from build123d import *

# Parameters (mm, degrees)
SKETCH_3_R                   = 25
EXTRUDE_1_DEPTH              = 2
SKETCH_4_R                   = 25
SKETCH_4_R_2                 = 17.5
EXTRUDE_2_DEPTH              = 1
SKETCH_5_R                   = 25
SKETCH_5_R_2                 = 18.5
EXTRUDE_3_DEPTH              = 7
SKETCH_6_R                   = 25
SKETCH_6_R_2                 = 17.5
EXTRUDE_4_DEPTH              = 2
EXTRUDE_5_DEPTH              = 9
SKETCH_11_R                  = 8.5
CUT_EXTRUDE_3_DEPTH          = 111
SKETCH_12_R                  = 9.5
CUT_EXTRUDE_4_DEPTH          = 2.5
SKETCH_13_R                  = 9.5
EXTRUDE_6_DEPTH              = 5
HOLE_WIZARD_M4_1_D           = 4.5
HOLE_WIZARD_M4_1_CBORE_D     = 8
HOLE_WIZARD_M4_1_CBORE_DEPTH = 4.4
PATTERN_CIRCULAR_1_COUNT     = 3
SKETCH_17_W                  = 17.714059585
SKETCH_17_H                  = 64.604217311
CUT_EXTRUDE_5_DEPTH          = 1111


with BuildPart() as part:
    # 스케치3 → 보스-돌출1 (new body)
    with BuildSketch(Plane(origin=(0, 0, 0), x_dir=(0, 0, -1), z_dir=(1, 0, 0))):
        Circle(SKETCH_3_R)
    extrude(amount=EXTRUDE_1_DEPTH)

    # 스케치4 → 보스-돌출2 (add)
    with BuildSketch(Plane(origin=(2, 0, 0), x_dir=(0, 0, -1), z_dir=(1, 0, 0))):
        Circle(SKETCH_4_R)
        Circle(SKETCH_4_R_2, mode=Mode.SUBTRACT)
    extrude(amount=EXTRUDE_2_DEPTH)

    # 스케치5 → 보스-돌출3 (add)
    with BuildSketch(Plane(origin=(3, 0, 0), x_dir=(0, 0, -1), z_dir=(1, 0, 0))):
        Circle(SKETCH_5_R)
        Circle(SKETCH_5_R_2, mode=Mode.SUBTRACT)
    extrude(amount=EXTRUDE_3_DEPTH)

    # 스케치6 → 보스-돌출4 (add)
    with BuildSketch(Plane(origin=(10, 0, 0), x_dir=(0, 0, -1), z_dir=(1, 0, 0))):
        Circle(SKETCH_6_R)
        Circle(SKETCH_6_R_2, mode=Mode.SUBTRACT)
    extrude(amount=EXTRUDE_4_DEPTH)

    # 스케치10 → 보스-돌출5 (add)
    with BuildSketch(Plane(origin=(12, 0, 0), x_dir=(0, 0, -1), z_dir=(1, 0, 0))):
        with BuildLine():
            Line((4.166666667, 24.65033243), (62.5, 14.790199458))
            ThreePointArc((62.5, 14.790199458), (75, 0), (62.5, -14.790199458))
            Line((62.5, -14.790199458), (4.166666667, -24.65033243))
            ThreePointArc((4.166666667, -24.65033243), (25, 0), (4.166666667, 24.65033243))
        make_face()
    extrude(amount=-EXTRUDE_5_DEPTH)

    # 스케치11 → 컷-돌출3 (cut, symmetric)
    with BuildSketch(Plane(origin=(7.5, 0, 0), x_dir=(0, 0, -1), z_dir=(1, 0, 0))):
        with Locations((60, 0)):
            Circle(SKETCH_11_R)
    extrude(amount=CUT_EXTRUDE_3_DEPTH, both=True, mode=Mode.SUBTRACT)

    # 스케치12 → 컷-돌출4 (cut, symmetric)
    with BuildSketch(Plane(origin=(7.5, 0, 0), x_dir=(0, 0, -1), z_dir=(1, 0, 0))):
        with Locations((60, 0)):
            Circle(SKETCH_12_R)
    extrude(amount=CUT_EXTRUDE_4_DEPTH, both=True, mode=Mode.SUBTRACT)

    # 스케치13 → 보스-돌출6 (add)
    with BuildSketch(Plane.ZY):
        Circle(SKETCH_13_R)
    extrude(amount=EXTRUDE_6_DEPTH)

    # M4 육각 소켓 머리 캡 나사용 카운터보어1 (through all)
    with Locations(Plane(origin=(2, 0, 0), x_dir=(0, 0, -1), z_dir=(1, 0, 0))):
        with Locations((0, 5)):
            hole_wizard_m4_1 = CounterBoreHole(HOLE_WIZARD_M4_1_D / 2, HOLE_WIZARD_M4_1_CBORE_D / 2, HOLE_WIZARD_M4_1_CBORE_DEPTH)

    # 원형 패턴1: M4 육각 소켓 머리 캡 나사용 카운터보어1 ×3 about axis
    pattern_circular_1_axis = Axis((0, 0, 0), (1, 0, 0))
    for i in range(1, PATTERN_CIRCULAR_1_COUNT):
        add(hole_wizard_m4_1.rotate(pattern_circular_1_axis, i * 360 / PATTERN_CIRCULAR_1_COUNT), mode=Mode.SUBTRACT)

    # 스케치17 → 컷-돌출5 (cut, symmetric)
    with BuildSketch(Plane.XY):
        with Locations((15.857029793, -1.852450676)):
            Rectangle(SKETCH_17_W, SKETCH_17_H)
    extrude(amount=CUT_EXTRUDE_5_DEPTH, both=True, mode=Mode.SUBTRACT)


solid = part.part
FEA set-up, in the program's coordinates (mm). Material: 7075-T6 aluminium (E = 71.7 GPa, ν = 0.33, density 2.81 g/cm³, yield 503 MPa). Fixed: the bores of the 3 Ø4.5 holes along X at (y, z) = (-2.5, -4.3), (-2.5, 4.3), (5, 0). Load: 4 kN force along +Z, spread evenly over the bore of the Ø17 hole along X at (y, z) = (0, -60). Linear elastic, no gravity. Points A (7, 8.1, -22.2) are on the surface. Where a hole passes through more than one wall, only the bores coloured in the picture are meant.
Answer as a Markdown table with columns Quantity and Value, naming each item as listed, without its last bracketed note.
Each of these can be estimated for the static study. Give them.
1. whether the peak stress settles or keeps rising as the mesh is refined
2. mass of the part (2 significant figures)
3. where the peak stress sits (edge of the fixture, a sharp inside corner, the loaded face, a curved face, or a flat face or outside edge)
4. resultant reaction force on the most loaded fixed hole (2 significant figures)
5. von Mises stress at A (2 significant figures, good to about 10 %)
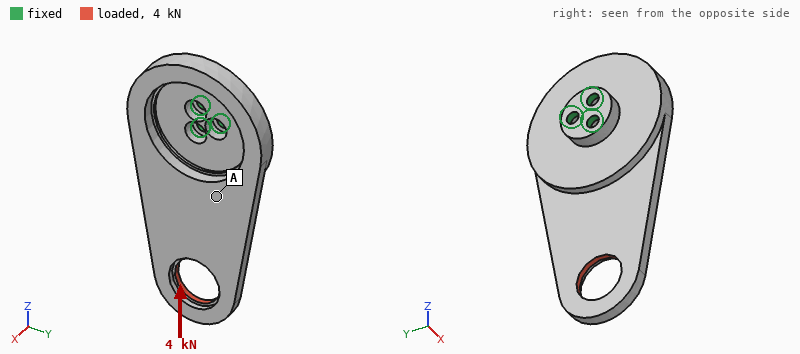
| Quantity | Value |
|---|---|
| whether the peak stress settles or keeps rising as the mesh is refined | keeps rising |
| mass of the part | 43 g |
| where the peak stress sits | edge of the fixture |
| resultant reaction force on the most loaded fixed hole | 2.5 kN |
| von Mises stress at A | 28 MPa |
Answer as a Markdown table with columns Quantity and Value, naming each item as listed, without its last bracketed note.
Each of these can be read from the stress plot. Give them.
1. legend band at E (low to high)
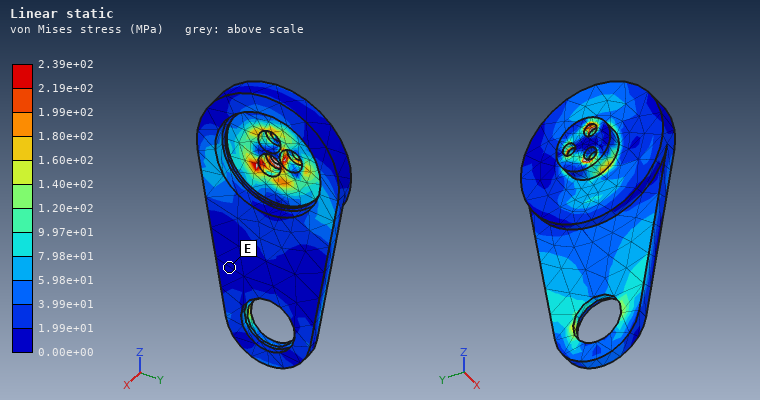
| Quantity | Value |
|---|---|
| legend band at E | 0.00e+00 to 1.99e+01 MPa |
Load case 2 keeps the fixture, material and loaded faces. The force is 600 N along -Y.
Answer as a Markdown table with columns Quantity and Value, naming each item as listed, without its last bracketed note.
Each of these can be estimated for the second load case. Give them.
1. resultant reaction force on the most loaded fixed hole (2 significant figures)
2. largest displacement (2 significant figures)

| Quantity | Value |
|---|---|
| resultant reaction force on the most loaded fixed hole | 2.0 kN |
| largest displacement | 0.19 mm |
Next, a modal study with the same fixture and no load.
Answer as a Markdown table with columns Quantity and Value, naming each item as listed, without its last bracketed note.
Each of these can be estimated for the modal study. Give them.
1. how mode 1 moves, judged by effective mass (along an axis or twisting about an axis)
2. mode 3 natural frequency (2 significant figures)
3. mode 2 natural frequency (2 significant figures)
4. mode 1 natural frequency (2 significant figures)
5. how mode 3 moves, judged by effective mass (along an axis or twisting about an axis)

| Quantity | Value |
|---|---|
| how mode 1 moves, judged by effective mass | along X |
| mode 3 natural frequency | 3100 Hz |
| mode 2 natural frequency | 2400 Hz |
| mode 1 natural frequency | 890 Hz |
| how mode 3 moves, judged by effective mass | along Y |
